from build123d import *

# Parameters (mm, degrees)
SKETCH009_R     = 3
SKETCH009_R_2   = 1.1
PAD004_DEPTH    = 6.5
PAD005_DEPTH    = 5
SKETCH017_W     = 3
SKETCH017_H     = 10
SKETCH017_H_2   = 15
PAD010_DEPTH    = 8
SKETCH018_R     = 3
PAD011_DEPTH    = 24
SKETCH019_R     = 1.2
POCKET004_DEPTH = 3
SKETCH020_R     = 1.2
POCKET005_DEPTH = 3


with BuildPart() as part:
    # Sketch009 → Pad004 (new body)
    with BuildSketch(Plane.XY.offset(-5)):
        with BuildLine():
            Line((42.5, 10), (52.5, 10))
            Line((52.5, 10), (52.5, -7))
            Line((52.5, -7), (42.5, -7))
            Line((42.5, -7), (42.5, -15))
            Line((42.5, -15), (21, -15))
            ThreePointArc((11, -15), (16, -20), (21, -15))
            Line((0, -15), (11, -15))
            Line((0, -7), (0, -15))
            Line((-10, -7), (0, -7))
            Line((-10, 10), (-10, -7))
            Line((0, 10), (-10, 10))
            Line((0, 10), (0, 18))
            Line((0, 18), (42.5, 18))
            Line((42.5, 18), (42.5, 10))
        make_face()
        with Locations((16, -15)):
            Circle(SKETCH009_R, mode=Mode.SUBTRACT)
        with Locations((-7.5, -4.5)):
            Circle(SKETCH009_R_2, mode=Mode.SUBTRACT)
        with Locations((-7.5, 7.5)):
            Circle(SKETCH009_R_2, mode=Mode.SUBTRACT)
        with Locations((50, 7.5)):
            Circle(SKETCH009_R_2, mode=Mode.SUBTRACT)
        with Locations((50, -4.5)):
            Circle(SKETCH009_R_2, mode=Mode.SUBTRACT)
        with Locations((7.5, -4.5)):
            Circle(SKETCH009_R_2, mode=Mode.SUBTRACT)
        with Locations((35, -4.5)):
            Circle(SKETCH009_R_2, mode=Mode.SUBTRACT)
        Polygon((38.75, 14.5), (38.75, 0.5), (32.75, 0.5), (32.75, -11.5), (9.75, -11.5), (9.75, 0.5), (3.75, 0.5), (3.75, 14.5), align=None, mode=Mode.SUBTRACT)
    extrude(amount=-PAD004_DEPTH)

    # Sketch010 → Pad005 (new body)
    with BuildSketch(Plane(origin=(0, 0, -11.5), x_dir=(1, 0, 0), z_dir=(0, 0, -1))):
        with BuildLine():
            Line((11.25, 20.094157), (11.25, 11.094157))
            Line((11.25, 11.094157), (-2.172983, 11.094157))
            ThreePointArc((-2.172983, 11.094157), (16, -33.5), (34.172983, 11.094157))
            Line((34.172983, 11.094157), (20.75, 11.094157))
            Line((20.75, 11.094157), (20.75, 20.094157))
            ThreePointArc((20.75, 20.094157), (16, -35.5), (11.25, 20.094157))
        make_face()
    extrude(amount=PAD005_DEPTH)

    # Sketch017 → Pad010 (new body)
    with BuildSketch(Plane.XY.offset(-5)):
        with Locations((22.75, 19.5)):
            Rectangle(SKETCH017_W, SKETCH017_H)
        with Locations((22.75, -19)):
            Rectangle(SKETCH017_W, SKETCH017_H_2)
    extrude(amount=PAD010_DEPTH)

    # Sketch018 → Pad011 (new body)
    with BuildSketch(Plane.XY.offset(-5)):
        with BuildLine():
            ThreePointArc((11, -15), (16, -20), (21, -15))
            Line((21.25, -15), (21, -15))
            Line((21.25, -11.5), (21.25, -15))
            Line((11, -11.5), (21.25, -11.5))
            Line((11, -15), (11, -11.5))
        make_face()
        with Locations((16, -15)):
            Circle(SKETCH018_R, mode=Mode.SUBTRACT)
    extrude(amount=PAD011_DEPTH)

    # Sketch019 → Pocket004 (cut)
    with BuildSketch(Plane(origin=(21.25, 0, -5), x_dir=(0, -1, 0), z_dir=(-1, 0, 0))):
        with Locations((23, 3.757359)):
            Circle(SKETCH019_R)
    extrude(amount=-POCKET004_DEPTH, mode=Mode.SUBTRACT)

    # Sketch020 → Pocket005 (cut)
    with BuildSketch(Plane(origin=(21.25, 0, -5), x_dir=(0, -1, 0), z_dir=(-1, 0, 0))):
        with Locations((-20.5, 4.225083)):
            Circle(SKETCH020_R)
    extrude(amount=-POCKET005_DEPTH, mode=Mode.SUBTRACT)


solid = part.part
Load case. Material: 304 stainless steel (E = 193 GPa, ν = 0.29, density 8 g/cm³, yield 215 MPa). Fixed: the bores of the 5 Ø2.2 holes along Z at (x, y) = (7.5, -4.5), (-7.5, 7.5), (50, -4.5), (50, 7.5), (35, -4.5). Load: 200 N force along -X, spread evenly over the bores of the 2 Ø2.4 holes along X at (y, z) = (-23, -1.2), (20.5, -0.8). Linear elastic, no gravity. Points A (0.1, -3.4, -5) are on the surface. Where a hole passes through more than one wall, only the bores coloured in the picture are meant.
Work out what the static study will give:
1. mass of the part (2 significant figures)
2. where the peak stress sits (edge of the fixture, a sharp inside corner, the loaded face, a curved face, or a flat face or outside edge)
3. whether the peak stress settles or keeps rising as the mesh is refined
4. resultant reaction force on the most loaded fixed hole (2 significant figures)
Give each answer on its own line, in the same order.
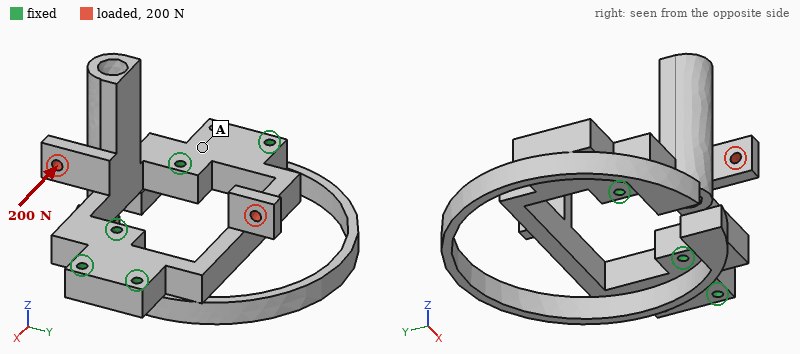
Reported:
81 g
a sharp inside corner
keeps rising
67 N
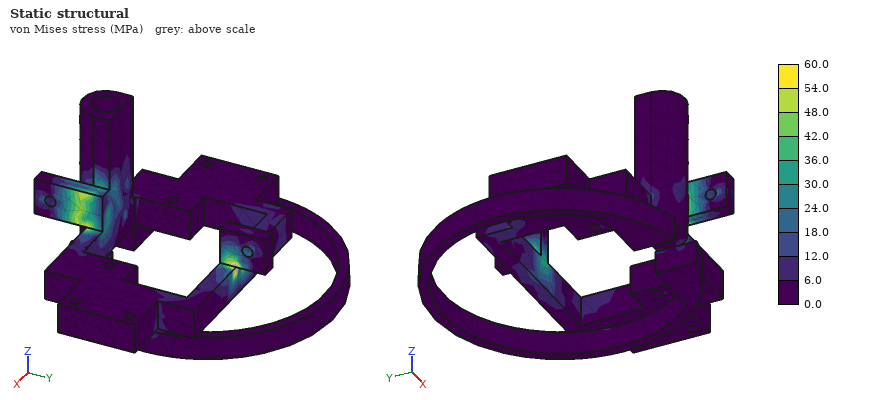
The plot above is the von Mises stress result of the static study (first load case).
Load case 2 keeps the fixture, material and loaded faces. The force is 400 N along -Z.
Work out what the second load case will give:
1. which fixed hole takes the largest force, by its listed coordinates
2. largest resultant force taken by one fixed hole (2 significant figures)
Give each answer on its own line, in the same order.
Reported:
(35, -4.5)
210 N
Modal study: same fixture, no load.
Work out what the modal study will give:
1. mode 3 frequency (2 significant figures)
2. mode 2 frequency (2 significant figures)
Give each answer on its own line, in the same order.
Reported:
3900 Hz
3300 Hz
